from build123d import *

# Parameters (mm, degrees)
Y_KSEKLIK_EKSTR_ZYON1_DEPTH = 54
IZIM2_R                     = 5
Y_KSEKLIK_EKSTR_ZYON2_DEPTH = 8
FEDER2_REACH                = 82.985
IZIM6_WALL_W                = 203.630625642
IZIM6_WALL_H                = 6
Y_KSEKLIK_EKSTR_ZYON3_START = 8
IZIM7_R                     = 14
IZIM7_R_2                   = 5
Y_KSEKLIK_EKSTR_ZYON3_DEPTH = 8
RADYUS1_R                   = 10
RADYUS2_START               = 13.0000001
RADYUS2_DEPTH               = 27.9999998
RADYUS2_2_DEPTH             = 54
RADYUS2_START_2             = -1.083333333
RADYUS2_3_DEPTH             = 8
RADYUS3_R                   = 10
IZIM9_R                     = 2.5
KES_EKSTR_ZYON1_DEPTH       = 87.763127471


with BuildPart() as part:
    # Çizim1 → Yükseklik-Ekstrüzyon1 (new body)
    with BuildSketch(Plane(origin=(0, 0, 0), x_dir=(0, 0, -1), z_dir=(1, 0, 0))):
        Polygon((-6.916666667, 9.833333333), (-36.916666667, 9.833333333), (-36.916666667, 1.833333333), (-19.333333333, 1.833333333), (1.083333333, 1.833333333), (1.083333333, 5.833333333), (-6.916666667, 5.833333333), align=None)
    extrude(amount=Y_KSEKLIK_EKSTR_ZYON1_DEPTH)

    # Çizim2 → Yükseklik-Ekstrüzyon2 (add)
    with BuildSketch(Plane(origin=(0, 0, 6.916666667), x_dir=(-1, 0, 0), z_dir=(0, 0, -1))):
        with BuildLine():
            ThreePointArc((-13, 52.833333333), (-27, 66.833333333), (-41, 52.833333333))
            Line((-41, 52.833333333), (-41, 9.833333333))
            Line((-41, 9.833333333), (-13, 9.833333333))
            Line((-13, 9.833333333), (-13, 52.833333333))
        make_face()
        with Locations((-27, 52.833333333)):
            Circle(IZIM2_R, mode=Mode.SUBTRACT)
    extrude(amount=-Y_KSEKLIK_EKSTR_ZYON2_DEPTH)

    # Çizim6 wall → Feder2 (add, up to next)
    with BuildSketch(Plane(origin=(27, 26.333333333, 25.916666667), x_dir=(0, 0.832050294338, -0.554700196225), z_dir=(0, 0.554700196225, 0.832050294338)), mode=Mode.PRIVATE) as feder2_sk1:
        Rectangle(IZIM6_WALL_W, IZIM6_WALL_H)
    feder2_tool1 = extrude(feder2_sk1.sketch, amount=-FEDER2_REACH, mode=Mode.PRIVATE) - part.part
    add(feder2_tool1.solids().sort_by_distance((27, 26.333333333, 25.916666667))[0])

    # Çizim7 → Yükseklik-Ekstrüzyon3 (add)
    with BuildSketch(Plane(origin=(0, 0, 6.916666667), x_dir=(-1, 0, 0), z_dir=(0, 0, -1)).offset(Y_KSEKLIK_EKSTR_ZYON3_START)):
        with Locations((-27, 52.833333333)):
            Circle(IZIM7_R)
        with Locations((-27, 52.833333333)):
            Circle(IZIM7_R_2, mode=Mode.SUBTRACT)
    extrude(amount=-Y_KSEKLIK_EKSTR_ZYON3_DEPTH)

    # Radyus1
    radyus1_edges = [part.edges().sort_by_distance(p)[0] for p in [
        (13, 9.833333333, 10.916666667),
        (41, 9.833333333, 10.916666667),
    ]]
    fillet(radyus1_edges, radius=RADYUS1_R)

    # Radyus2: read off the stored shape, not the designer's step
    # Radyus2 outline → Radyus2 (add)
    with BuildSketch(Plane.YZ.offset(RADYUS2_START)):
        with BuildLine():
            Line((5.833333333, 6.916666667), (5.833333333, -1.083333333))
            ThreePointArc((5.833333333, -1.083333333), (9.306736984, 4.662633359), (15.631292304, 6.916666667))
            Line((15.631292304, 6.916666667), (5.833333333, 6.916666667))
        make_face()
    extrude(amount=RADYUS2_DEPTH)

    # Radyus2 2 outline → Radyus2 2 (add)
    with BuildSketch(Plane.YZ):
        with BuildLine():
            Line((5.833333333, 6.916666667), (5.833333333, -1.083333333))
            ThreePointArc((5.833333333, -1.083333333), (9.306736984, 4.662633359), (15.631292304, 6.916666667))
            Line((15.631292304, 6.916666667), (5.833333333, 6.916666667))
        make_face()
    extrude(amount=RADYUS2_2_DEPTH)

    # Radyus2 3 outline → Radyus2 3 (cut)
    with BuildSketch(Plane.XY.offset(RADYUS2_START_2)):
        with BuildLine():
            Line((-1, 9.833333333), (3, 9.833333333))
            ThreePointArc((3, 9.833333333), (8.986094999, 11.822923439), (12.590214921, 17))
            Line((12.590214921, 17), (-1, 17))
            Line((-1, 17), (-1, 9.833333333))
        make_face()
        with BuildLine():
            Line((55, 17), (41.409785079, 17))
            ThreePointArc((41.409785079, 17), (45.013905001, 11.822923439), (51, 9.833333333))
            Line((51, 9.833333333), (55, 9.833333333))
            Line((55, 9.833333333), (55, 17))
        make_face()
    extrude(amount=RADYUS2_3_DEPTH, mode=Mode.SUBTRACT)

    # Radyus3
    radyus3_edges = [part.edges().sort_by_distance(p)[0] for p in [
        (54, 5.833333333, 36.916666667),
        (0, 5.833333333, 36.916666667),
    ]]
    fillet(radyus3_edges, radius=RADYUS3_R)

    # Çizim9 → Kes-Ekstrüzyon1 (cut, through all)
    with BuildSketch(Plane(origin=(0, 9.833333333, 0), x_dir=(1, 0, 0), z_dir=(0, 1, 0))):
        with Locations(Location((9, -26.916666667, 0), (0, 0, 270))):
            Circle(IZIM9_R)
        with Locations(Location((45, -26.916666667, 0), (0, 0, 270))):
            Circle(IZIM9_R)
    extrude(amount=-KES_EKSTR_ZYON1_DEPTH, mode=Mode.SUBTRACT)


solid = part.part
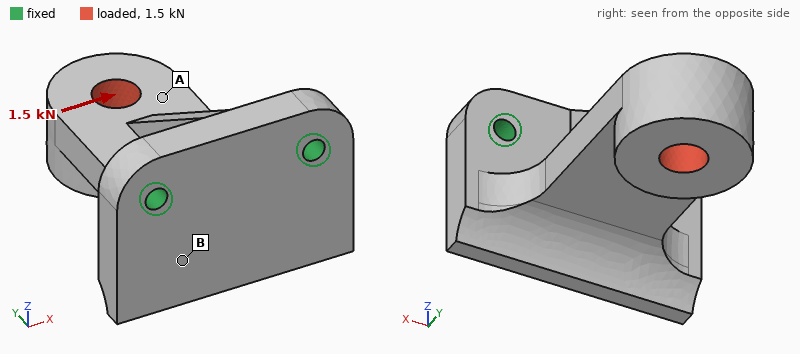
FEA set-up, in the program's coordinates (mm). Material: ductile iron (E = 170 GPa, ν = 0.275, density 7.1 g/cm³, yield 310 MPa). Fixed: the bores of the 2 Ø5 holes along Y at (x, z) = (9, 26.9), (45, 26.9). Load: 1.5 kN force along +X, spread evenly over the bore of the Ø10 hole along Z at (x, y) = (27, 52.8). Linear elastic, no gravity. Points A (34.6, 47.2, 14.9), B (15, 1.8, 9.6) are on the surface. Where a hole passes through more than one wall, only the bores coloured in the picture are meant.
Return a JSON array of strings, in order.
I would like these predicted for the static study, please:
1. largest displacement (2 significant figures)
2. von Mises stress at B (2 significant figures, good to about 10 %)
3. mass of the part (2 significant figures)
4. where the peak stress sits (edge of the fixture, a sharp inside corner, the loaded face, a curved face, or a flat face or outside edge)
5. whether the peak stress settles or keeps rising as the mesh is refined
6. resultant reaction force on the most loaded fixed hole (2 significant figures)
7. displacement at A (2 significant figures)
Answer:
["63 µm", "29 MPa", "240 g", "edge of the fixture", "keeps rising", "2.2 kN", "36 µm"]
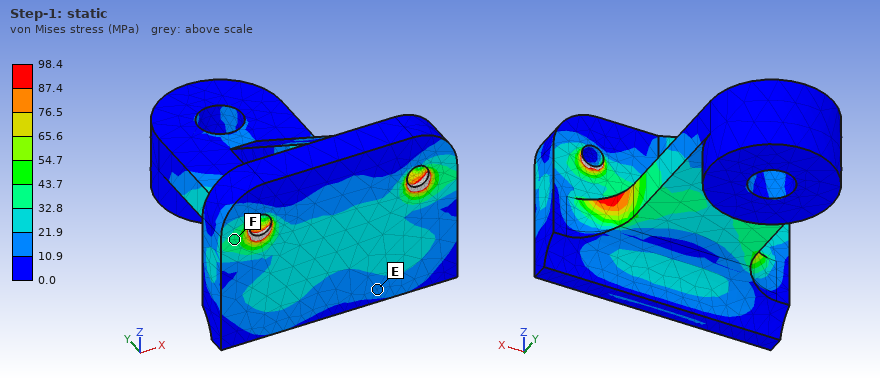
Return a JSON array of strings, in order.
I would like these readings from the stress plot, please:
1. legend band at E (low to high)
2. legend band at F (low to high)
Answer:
["10.9 to 21.9 MPa", "32.8 to 43.7 MPa"]
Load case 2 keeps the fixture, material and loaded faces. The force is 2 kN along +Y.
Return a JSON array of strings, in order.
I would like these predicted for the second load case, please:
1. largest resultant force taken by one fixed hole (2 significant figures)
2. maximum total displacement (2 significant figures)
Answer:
["1.0 kN", "77 µm"]
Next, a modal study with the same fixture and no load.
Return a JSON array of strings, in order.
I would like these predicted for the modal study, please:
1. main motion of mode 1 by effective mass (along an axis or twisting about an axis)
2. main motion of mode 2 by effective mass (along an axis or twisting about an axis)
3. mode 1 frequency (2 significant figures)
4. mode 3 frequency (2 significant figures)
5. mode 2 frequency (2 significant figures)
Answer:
["along Z", "along X", "1900 Hz", "6800 Hz", "3300 Hz"]
